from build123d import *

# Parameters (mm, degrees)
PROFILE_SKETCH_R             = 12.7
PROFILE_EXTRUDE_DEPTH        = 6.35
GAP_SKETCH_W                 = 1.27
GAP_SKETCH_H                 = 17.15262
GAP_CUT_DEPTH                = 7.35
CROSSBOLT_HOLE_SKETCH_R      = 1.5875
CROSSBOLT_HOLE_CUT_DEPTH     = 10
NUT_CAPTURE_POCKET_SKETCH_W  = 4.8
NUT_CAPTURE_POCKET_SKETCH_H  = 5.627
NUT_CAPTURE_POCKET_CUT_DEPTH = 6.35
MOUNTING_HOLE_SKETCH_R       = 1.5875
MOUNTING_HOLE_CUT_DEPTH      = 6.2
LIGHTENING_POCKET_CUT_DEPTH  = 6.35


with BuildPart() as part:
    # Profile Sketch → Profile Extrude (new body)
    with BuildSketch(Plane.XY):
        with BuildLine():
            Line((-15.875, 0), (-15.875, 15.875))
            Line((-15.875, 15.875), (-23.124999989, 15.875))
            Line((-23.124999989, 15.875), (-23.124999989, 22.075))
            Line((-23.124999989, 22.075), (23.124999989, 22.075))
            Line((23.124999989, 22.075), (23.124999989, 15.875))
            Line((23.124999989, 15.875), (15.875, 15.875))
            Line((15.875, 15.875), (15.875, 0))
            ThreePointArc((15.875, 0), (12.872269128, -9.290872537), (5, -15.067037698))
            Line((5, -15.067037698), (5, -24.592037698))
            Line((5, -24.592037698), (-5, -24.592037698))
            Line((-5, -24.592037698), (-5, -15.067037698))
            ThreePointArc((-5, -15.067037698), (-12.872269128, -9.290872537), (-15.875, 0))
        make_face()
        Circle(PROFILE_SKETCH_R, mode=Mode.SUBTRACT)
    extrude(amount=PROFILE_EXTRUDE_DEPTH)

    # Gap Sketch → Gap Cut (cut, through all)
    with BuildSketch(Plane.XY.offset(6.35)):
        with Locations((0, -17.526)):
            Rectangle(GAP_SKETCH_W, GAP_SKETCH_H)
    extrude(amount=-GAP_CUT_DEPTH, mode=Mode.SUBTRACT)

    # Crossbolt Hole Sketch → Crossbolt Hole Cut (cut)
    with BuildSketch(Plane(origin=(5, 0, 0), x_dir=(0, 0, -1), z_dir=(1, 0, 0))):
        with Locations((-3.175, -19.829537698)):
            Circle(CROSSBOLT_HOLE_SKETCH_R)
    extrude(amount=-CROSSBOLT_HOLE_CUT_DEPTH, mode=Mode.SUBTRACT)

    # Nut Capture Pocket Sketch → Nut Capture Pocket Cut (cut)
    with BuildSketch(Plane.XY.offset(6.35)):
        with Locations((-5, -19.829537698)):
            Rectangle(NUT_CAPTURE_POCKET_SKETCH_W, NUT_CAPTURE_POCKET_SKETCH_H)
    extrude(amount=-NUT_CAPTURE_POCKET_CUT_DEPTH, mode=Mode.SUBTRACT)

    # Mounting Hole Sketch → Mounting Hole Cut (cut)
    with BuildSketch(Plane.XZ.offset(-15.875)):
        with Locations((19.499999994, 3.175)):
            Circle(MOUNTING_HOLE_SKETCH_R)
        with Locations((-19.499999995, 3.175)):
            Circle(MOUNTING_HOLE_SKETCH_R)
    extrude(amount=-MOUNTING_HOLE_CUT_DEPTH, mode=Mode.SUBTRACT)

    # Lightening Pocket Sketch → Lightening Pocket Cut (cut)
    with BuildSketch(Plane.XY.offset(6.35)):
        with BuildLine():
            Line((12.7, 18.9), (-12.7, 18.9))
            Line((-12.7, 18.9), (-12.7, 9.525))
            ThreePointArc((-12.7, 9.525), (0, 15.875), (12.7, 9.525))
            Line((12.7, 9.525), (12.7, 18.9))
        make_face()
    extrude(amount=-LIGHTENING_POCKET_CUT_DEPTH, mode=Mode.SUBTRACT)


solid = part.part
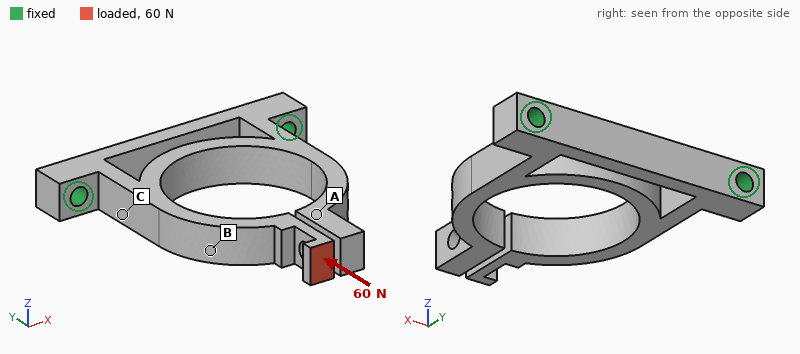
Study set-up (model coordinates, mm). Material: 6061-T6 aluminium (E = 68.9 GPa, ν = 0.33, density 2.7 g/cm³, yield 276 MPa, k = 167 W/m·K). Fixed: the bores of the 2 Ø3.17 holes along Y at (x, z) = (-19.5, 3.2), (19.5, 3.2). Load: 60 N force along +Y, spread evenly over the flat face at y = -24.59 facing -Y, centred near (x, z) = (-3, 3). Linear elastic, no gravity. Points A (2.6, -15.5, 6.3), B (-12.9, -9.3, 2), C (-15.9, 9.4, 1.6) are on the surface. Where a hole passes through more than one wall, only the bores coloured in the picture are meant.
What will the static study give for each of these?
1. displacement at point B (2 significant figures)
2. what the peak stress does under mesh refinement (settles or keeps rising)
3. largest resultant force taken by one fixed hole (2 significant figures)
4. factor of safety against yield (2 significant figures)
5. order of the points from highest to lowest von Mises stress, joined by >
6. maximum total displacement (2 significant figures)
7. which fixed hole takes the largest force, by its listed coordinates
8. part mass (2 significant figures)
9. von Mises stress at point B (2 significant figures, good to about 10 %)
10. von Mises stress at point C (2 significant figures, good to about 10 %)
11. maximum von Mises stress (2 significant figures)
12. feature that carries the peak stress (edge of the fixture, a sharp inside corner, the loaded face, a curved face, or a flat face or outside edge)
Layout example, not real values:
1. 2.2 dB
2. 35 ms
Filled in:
1. 0.11 mm
2. settles
3. 42 N
4. 3.8
5. B > C > A
6. 0.33 mm
7. (-19.5, 3.2)
8. 10 g
9. 43 MPa
10. 24 MPa
11. 72 MPa
12. a curved face
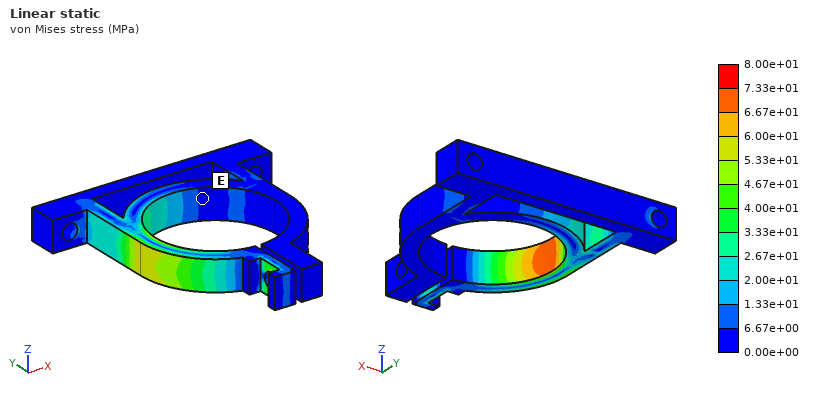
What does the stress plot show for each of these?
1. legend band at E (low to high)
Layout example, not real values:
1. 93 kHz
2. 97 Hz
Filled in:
1. 0.00e+00 to 6.67e+00 MPa
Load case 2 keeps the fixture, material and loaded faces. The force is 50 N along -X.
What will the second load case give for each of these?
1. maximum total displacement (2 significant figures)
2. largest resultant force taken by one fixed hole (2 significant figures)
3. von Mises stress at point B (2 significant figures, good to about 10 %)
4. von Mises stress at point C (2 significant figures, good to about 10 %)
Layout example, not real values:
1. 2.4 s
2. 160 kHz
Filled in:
1. 0.76 mm
2. 53 N
3. 71 MPa
4. 66 MPa
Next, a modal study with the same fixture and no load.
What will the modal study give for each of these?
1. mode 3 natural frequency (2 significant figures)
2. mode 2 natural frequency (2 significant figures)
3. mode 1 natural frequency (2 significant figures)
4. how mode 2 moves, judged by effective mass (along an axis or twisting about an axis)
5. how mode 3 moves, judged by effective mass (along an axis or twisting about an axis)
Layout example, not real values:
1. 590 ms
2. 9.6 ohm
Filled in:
1. 2000 Hz
2. 1800 Hz
3. 1500 Hz
4. along X
5. along Z
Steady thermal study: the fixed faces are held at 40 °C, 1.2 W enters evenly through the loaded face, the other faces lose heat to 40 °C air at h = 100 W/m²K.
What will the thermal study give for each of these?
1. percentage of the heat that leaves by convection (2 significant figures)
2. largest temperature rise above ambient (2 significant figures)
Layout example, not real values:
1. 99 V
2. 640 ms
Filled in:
1. 49 %
2. 14 K
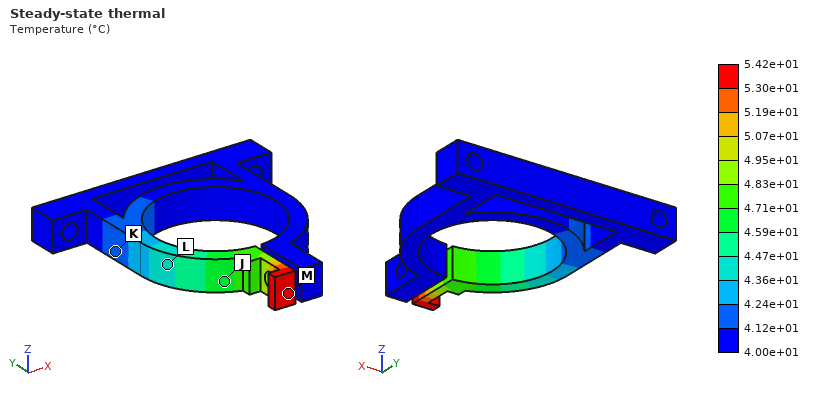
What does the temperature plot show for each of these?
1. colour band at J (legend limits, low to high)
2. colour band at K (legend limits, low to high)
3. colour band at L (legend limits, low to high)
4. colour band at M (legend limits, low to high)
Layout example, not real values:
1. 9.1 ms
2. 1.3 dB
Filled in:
1. 4.59e+01 to 4.71e+01 °C
2. 4.12e+01 to 4.24e+01 °C
3. 4.36e+01 to 4.47e+01 °C
4. 5.30e+01 to 5.42e+01 °C
